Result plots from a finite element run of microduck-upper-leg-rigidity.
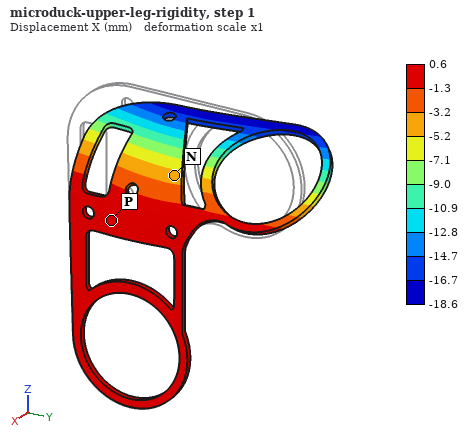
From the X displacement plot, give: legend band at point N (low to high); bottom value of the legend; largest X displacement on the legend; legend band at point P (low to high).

-5.2 to -3.2 mm
-18.6 mm
0.6 mm
-1.3 to 0.6 mm
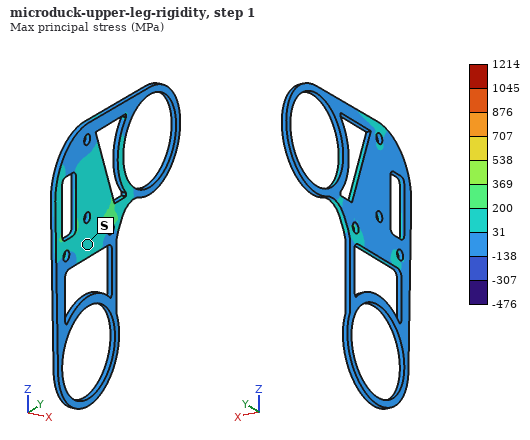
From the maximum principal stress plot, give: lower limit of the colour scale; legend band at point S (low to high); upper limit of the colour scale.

-476 MPa
31 to 200 MPa
1214 MPa
